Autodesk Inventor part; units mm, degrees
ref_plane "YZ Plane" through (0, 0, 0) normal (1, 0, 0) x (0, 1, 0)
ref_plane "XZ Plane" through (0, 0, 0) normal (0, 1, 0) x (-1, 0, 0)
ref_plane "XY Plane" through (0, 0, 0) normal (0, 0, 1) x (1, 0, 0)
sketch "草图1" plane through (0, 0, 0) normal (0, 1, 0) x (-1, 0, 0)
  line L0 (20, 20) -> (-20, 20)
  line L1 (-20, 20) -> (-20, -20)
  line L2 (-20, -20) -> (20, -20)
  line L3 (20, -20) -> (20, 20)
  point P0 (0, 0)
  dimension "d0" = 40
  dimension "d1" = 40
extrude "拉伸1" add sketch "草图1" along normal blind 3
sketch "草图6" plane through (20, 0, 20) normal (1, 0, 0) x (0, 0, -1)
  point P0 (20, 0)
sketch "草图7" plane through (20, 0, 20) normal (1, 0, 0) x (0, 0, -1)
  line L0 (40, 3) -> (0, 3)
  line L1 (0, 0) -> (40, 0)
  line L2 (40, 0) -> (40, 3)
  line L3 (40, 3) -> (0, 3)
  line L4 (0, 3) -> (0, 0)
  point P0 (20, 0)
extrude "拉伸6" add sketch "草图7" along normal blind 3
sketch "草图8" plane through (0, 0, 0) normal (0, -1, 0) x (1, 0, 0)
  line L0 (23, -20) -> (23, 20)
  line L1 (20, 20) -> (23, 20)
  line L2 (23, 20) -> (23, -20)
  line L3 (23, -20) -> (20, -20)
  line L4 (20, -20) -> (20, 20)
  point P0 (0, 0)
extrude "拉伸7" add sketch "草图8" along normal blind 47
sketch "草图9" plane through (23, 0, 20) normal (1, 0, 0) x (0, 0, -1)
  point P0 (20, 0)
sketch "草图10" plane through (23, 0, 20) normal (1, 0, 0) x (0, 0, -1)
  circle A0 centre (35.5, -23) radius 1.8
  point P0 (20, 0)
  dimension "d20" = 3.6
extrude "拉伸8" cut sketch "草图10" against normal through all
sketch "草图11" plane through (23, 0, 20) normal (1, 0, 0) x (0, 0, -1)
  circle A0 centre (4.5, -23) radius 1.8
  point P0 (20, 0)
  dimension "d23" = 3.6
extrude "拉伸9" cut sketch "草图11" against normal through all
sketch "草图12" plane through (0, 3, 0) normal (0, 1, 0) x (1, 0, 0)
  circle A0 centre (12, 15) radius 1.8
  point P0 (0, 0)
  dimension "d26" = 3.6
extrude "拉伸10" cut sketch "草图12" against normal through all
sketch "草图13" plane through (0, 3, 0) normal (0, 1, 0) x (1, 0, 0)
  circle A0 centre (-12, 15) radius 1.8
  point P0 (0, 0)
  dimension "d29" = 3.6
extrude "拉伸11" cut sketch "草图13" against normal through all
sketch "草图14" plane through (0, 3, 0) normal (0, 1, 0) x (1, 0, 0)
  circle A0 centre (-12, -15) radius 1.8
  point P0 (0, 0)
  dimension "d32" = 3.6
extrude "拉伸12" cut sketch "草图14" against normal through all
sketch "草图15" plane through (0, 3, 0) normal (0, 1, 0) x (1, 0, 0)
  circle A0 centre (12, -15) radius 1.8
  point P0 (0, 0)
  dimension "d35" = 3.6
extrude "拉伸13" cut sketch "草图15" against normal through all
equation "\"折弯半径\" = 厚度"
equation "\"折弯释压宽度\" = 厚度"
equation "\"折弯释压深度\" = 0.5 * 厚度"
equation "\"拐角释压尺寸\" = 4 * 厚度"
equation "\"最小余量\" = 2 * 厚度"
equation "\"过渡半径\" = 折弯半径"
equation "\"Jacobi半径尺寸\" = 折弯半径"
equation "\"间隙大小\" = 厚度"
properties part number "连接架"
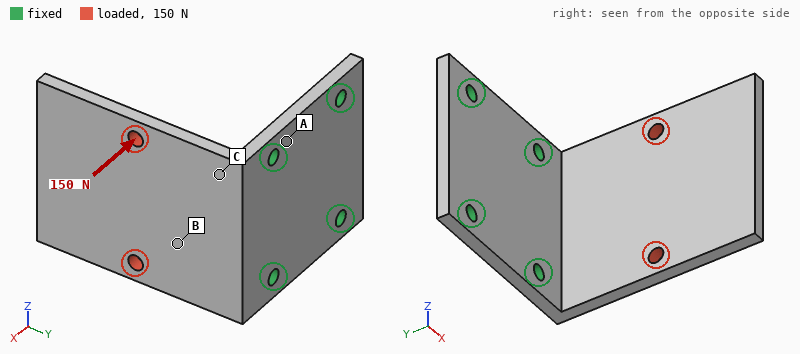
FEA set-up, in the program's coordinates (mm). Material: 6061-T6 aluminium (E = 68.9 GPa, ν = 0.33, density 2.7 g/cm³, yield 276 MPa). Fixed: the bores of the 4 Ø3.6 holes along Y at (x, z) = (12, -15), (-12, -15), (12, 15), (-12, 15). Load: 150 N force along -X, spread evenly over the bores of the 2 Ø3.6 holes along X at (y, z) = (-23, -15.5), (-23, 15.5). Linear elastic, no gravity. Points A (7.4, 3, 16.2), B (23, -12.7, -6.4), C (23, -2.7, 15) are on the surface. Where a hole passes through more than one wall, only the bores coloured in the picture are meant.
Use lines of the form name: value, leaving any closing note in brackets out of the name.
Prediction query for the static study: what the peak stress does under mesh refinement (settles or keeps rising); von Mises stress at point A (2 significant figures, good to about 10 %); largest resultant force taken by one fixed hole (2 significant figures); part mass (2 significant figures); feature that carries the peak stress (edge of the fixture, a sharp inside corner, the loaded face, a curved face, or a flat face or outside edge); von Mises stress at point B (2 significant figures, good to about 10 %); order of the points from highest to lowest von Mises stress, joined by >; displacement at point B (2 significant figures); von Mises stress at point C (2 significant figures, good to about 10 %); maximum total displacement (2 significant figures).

what the peak stress does under mesh refinement: keeps rising
von Mises stress at point A: 8.0 MPa
largest resultant force taken by one fixed hole: 59 N
part mass: 29 g
feature that carries the peak stress: edge of the fixture
von Mises stress at point B: 22 MPa
order of the points from highest to lowest von Mises stress, joined by >: C > B > A
displacement at point B: 0.12 mm
von Mises stress at point C: 46 MPa
maximum total displacement: 0.50 mm
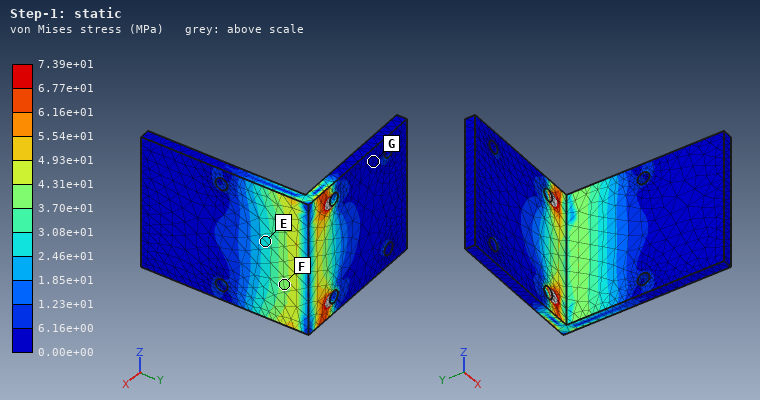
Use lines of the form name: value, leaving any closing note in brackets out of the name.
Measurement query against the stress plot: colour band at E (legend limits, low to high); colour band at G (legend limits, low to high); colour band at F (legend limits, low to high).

colour band at E: 2.46e+01 to 3.08e+01 MPa
colour band at G: 0.00e+00 to 6.16e+00 MPa
colour band at F: 3.70e+01 to 4.31e+01 MPa
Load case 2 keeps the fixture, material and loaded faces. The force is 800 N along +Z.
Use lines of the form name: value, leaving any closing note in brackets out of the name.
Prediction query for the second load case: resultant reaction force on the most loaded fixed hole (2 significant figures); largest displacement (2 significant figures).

resultant reaction force on the most loaded fixed hole: 790 N
largest displacement: 0.20 mm
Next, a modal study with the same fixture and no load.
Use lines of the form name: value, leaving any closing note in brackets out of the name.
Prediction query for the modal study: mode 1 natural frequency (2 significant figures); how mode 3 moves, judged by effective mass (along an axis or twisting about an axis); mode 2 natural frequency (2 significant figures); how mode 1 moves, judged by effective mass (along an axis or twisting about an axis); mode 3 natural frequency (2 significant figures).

mode 1 natural frequency: 810 Hz
how mode 3 moves, judged by effective mass: along Z
mode 2 natural frequency: 2500 Hz
how mode 1 moves, judged by effective mass: along X
mode 3 natural frequency: 3600 Hz
